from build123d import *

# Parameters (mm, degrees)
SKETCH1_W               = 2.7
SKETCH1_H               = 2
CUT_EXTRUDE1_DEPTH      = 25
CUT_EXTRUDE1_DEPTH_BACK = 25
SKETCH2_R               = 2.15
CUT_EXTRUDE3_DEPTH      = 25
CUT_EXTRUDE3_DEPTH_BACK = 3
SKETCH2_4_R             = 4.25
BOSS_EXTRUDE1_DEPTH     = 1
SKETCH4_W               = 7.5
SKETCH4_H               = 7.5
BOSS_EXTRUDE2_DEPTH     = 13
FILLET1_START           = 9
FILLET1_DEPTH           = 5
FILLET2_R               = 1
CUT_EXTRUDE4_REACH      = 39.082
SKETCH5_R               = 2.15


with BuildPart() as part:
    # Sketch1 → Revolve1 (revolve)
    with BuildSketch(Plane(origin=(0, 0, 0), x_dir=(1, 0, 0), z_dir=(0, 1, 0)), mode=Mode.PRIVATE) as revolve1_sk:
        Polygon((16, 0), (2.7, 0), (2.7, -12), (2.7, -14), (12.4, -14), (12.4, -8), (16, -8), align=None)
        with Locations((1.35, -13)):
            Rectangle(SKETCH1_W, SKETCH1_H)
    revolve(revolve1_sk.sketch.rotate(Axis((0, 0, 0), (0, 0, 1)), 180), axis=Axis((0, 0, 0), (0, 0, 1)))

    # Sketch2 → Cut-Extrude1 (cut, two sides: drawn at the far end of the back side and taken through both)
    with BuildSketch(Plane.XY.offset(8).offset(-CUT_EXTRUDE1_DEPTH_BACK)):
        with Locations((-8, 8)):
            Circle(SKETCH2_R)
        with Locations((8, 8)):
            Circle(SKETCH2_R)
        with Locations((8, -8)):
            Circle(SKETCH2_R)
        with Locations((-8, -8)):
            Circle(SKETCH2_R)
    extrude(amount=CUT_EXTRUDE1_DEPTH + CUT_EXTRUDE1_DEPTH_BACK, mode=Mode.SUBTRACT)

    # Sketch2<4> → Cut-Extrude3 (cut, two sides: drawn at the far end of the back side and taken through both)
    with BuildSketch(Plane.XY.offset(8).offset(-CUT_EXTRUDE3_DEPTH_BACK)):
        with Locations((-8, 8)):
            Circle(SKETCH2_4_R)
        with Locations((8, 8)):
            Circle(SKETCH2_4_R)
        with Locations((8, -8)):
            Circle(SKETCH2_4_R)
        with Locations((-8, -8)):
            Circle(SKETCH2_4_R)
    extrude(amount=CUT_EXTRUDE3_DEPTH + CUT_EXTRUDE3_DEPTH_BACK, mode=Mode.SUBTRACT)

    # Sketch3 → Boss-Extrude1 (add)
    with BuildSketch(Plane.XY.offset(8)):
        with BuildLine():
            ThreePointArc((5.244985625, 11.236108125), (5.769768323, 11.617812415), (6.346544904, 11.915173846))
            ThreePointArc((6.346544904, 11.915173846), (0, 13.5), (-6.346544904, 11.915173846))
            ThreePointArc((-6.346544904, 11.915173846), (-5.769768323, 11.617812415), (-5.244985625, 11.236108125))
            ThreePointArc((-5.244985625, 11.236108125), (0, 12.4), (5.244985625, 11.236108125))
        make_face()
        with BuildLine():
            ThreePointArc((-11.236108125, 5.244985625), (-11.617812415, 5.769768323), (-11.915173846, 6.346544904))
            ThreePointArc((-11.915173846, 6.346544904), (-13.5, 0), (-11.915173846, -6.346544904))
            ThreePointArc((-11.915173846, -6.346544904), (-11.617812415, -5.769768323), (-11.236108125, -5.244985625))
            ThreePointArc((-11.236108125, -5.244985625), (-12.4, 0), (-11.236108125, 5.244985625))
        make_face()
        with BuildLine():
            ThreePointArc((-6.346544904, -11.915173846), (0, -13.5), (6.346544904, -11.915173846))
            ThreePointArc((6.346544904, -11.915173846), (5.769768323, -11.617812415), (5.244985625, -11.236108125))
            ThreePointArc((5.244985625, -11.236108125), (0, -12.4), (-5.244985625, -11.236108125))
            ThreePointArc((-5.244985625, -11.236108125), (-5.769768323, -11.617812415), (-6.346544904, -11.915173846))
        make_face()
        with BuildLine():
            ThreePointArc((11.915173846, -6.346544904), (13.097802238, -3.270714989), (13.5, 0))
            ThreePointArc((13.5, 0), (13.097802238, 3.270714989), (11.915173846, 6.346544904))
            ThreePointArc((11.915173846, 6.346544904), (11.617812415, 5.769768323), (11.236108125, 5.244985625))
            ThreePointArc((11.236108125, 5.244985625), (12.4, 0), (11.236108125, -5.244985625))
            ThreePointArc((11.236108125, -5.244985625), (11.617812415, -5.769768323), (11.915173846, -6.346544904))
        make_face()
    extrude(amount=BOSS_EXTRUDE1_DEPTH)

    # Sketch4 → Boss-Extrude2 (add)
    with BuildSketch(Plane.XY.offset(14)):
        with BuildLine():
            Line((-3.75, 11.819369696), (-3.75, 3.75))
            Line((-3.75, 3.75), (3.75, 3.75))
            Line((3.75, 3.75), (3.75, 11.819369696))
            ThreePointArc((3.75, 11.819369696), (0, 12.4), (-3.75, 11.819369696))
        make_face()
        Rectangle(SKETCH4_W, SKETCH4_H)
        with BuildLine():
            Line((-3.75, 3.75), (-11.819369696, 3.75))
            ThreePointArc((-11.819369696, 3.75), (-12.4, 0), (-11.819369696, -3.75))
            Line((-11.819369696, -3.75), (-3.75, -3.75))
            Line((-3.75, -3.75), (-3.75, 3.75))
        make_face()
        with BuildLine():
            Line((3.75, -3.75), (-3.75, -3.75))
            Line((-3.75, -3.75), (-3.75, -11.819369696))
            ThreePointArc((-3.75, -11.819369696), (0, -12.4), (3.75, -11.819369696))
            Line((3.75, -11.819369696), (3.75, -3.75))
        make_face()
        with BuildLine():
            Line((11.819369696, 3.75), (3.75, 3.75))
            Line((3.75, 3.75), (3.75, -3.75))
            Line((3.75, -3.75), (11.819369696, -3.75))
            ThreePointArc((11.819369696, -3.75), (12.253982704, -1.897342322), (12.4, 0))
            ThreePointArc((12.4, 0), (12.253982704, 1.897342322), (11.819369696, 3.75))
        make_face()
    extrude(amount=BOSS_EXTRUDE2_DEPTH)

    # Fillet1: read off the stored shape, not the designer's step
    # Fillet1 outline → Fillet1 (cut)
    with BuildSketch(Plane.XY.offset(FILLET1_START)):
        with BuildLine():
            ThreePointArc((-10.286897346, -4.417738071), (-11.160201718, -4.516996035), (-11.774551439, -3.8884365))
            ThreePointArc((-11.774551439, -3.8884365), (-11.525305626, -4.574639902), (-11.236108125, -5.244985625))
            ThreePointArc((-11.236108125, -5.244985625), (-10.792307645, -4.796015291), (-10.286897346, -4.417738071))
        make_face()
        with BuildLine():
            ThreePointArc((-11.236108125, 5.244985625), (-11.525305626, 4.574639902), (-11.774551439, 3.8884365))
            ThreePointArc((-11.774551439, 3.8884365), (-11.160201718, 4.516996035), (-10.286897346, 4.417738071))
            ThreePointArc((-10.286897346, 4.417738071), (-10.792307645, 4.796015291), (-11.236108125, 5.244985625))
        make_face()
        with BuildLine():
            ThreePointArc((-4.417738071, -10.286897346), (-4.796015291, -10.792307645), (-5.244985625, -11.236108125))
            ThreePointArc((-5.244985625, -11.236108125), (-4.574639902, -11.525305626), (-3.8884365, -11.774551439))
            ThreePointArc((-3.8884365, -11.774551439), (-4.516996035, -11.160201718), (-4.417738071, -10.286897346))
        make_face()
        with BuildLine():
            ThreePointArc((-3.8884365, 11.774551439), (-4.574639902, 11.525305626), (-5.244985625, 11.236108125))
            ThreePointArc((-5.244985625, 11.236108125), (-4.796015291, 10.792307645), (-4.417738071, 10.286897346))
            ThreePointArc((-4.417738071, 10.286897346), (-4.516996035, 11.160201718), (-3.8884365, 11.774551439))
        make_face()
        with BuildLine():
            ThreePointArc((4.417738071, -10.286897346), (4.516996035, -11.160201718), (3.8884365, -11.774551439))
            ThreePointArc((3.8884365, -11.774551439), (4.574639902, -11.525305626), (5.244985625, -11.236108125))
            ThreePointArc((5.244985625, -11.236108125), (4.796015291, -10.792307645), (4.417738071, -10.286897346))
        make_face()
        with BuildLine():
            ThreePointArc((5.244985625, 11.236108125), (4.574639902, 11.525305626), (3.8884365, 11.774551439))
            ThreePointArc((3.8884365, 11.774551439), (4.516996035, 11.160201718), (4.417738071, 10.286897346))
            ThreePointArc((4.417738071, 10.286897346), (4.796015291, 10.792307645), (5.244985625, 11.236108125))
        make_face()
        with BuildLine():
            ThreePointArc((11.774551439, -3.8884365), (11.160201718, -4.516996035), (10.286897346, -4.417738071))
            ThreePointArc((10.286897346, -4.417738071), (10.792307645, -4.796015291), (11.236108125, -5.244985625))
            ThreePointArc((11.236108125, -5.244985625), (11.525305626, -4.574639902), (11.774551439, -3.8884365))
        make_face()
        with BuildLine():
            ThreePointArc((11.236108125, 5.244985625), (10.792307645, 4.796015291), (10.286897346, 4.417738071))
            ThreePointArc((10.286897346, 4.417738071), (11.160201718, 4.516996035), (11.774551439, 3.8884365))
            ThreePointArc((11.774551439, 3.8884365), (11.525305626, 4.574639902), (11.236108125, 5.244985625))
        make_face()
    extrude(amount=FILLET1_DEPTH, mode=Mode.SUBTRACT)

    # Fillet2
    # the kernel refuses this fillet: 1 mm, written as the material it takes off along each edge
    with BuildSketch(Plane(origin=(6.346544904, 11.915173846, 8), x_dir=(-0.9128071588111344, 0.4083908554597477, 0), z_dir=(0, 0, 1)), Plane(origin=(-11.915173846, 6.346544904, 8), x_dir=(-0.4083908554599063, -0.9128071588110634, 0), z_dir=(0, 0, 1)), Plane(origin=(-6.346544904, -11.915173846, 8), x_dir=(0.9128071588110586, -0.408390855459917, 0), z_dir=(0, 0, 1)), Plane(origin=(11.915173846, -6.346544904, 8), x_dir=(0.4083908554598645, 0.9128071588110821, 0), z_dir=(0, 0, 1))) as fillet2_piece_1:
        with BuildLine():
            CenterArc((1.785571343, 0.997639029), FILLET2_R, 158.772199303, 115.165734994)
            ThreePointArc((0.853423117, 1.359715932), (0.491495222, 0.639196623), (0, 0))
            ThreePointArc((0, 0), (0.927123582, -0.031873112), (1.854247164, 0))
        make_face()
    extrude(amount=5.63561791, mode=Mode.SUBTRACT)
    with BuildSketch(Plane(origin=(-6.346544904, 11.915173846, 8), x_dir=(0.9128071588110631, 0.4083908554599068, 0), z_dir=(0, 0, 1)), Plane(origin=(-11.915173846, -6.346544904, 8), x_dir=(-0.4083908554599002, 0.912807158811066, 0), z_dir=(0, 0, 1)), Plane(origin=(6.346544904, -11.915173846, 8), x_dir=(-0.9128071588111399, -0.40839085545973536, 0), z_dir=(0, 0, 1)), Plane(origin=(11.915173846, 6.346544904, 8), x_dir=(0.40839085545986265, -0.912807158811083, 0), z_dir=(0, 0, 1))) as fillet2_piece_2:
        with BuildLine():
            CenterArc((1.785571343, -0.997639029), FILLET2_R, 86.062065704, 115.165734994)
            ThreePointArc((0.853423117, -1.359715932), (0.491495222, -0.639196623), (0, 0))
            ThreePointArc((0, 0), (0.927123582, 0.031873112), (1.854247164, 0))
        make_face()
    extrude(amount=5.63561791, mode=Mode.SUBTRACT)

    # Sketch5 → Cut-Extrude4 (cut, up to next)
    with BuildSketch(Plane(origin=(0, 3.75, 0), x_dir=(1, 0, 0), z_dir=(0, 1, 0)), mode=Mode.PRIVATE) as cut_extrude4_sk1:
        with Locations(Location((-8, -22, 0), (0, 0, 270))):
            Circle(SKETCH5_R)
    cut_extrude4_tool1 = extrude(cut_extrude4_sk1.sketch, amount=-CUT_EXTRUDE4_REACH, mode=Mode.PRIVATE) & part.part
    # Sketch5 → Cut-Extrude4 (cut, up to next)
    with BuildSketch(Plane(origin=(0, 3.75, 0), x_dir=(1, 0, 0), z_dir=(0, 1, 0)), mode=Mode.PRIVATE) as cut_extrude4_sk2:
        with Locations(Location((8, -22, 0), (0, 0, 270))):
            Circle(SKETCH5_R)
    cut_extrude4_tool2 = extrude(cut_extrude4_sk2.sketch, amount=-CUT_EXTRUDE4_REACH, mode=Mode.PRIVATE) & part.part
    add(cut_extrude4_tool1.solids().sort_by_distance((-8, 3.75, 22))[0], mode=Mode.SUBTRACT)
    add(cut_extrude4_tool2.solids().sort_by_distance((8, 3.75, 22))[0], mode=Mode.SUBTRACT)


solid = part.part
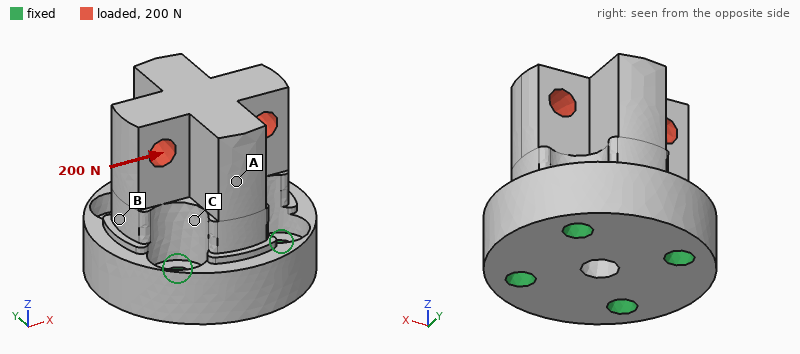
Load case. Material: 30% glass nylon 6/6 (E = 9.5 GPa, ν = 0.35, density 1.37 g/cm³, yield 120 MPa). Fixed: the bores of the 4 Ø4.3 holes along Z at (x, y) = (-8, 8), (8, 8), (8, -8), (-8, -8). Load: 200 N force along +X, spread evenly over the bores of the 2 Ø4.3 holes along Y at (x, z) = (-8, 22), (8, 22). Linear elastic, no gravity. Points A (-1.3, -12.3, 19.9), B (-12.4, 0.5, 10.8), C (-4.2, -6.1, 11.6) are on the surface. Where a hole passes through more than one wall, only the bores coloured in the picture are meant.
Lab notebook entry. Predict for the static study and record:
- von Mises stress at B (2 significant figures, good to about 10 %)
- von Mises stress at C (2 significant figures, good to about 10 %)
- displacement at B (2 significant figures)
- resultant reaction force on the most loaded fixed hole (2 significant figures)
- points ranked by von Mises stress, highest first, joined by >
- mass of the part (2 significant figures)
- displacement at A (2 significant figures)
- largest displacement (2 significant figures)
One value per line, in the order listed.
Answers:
3.0 MPa
1.7 MPa
6.5 µm
120 N
B > C > A
15 g
8.9 µm
16 µm
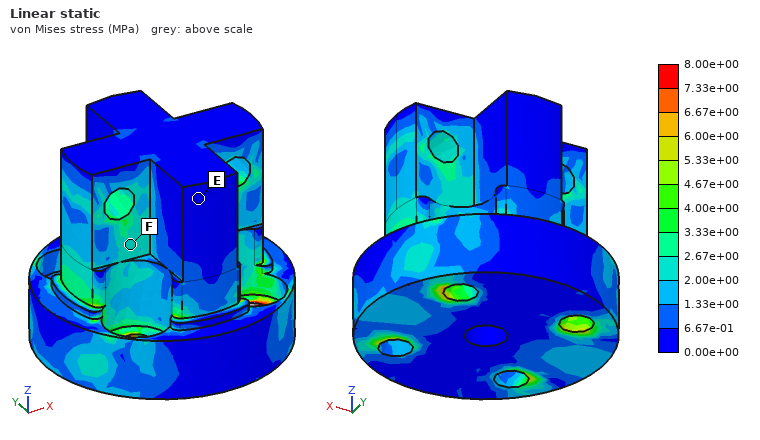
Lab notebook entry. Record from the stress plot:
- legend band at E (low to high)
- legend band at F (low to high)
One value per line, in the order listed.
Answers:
0.00e+00 to 6.67e-01 MPa
2.00e+00 to 2.67e+00 MPa
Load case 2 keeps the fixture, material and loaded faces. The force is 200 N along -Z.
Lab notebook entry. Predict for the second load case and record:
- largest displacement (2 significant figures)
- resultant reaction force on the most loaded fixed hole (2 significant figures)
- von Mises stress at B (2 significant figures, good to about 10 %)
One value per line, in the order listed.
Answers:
3.6 µm
52 N
1.3 MPa
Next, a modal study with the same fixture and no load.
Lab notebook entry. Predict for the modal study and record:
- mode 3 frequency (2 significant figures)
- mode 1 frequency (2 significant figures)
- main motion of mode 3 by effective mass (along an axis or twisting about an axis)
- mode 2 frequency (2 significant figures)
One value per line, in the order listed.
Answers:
13 kHz
8900 Hz
twisting about Z
8900 Hz
